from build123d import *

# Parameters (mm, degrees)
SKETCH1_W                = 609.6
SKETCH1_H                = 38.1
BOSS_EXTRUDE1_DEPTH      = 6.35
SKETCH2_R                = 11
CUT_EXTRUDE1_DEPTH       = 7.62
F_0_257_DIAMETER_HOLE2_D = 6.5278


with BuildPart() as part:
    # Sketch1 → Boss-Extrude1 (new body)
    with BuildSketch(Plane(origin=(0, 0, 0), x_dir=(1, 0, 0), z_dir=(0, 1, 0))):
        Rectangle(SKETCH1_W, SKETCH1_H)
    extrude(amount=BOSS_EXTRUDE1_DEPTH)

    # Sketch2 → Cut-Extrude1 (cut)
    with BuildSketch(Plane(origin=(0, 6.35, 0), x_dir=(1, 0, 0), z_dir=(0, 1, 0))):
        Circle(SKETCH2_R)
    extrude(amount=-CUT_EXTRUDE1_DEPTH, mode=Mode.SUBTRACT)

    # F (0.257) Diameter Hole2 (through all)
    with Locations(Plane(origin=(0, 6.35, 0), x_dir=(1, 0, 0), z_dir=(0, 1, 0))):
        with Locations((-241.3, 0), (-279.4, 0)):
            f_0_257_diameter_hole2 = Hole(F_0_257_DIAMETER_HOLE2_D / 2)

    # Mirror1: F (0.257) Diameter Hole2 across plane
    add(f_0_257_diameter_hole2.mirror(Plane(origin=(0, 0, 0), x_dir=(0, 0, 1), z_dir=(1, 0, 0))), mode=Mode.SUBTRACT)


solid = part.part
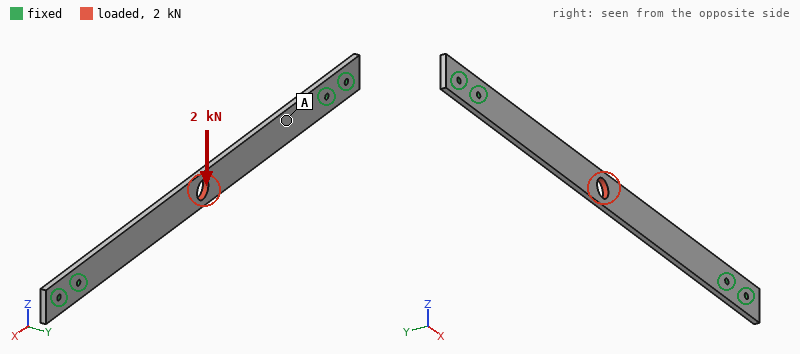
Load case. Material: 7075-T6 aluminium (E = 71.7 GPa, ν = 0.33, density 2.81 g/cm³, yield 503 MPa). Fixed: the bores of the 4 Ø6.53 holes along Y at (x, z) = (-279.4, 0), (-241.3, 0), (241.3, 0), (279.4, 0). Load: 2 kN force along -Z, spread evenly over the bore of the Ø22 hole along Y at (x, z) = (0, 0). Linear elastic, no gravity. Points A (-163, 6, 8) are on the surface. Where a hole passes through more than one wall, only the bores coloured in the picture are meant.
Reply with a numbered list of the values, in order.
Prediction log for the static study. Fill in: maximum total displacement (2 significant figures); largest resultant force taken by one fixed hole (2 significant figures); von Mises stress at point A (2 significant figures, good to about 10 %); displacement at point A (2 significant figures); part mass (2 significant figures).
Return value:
1. 0.73 mm
2. 3.3 kN
3. 13 MPa
4. 0.22 mm
5. 410 g
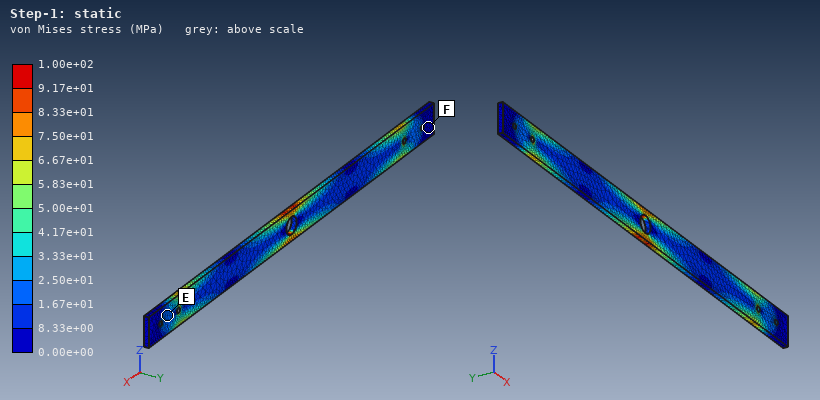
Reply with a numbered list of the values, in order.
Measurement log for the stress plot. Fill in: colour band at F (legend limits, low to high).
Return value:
1. 0.00e+00 to 8.33e+00 MPa
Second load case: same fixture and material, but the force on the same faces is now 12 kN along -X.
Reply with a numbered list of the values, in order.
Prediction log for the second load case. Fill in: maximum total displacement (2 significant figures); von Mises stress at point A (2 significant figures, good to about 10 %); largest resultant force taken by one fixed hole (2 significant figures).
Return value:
1. 87 µm
2. 25 MPa
3. 4.9 kN
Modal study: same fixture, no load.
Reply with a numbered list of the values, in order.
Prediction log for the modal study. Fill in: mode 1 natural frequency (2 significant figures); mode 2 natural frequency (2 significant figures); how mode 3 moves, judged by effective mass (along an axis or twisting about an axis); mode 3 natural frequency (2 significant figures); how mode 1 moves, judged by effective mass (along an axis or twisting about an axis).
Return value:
1. 140 Hz
2. 390 Hz
3. along Z
4. 740 Hz
5. along Y
